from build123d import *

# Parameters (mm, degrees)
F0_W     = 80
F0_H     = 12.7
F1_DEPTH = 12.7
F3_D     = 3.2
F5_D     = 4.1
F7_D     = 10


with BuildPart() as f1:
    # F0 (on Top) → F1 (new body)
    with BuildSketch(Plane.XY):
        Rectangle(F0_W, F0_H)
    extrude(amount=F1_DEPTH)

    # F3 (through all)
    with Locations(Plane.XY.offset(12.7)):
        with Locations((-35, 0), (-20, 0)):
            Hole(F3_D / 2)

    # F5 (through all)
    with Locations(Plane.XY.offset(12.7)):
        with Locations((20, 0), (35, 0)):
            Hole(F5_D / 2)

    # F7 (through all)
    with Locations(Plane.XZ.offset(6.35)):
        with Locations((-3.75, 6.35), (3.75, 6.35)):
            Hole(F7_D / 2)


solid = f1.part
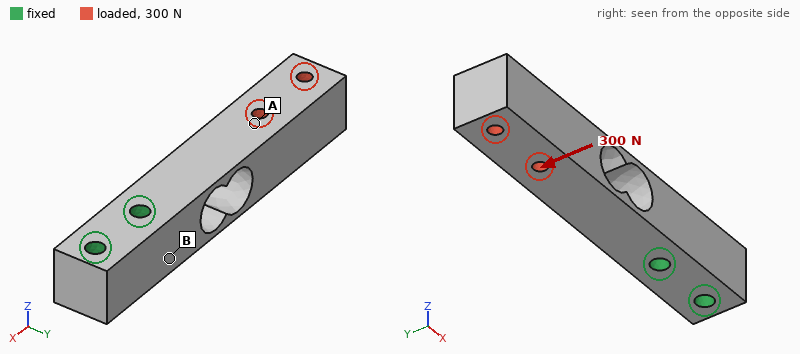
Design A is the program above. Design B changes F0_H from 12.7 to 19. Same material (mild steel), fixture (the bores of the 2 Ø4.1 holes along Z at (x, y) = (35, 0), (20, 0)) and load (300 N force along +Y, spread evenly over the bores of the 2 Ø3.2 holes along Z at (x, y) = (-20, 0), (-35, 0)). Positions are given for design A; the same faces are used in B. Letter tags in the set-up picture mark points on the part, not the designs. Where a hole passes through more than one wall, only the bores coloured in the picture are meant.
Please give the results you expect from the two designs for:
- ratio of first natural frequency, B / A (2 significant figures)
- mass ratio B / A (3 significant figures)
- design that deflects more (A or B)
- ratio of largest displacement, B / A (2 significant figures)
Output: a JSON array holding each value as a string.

["0.99", "1.52", "A", "0.35"]
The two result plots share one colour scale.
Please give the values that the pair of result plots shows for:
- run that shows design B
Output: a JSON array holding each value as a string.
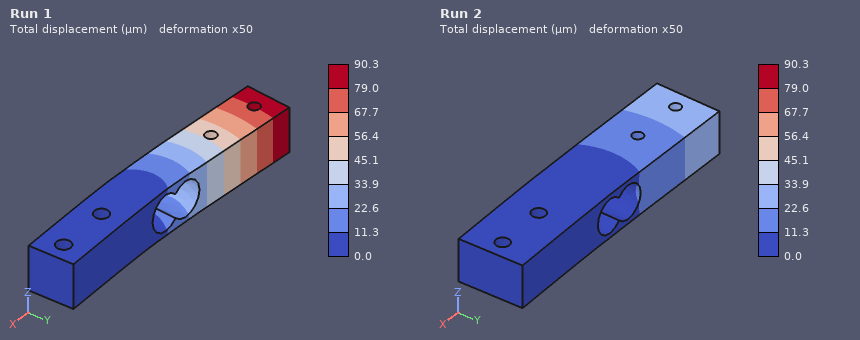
["Run 2"]
